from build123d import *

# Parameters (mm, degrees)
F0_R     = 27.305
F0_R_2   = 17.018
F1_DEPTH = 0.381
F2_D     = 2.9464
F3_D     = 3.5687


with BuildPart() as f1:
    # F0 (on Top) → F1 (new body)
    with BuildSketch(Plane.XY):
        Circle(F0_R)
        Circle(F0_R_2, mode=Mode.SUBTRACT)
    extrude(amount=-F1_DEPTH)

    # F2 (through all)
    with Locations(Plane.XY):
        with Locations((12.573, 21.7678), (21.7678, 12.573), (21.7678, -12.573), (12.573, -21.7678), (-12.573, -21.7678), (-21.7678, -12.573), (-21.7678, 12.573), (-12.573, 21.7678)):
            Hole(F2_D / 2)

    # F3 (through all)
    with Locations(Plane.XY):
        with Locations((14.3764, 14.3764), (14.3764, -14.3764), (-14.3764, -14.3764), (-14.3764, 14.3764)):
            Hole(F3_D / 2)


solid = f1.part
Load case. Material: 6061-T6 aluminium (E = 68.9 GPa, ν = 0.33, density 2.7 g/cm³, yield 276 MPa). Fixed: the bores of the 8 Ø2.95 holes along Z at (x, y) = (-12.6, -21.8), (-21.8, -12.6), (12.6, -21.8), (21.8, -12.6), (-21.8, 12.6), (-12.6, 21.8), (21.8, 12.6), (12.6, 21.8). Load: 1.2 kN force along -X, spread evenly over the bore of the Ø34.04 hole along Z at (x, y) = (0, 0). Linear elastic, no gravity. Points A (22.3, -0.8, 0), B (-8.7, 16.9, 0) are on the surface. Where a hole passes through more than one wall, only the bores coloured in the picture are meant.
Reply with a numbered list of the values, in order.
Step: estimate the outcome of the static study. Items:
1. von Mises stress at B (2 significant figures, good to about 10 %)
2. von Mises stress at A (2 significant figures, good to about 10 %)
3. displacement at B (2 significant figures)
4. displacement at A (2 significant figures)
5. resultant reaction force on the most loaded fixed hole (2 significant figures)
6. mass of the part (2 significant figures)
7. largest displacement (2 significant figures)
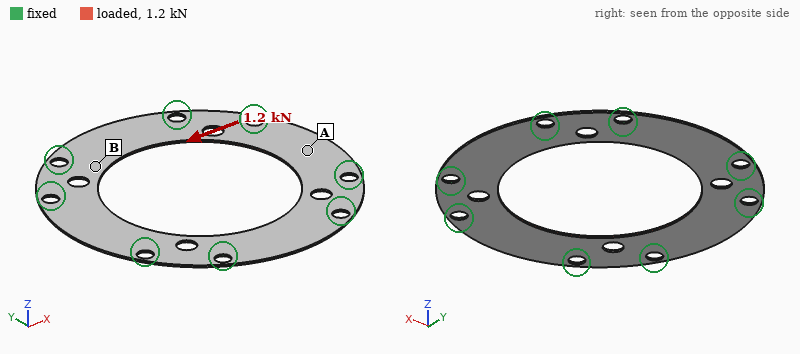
1. 49 MPa
2. 20 MPa
3. 5.5 µm
4. 16 µm
5. 180 N
6. 1.4 g
7. 18 µm
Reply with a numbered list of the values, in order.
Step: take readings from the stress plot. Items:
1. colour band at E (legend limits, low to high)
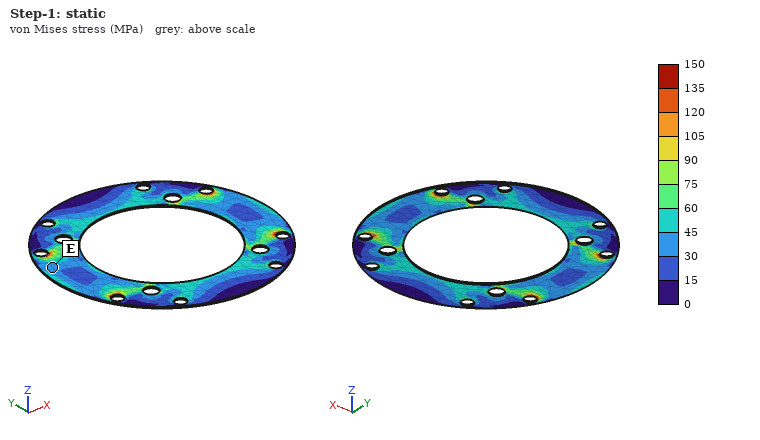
1. 30 to 45 MPa
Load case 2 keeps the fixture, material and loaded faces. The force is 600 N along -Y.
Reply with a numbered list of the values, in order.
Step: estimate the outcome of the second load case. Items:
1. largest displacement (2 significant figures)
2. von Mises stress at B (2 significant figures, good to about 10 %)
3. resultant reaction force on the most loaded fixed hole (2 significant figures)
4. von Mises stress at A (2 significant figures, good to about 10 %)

1. 8.9 µm
2. 19 MPa
3. 90 N
4. 10 MPa
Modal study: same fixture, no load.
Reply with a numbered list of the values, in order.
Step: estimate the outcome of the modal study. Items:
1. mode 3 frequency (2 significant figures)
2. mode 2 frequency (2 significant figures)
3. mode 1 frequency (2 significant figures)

1. 3600 Hz
2. 3600 Hz
3. 3600 Hz
